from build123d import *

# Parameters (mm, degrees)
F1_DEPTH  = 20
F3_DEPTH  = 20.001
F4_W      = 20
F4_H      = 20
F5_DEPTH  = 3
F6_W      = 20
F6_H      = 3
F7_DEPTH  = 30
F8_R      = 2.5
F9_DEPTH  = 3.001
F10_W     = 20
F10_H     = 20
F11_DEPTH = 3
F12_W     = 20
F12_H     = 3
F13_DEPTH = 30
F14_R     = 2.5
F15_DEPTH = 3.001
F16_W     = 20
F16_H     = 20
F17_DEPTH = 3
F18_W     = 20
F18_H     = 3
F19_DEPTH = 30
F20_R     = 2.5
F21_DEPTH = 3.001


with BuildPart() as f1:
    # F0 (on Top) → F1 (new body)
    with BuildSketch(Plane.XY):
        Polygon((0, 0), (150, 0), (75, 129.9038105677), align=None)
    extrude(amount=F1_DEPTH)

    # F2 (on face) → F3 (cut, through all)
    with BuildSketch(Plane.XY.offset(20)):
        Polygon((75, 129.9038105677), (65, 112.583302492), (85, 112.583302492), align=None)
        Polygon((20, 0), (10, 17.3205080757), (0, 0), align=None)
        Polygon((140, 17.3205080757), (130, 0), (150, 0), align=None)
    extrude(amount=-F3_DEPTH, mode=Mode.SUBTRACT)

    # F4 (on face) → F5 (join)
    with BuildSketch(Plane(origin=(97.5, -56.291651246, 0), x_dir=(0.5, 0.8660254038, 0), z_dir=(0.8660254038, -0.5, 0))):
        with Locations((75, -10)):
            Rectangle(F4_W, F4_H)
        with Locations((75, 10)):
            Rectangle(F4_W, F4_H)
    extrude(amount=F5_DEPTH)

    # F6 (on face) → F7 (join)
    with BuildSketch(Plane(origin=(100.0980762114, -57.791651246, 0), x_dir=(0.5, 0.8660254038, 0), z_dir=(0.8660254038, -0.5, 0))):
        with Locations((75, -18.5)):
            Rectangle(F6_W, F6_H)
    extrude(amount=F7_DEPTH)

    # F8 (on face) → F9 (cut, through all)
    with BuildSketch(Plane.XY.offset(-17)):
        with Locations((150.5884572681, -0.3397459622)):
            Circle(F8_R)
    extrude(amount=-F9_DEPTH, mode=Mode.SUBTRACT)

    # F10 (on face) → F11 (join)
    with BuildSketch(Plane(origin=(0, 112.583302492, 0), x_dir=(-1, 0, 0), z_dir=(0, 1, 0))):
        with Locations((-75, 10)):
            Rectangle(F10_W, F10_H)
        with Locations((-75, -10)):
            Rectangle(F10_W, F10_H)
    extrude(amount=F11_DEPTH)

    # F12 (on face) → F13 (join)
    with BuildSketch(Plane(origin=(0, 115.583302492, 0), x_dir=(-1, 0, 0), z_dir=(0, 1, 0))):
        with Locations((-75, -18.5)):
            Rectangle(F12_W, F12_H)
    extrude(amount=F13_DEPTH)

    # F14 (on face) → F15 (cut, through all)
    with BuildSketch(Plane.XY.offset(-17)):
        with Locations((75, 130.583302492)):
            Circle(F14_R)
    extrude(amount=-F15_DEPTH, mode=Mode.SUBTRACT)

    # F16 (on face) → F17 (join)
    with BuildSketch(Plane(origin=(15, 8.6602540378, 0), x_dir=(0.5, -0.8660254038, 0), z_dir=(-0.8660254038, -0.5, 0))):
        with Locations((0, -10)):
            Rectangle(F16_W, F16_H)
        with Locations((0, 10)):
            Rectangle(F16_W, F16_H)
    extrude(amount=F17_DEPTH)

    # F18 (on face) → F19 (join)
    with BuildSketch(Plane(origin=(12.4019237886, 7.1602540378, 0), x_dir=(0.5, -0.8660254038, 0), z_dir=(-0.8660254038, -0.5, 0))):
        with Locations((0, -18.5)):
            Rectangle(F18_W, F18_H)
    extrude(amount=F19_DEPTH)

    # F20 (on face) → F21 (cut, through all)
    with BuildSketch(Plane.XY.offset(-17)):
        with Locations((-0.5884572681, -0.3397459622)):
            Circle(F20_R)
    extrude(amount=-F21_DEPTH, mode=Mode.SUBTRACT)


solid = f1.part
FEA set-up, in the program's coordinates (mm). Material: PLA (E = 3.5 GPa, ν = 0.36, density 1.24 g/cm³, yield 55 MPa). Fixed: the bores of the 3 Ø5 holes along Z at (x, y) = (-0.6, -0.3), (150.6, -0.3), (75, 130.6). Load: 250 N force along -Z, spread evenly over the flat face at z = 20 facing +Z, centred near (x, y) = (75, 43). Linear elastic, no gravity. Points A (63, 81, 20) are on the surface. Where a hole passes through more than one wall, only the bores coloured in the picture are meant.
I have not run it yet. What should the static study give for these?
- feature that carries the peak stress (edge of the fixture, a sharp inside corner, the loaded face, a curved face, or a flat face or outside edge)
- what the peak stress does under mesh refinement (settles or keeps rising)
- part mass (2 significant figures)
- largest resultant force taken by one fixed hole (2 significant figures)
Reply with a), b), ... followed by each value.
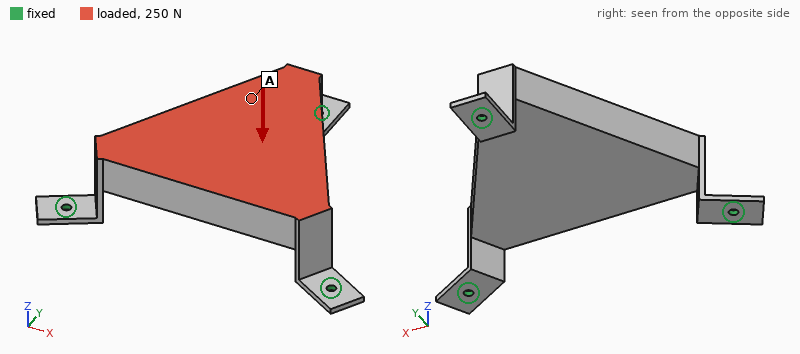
a) edge of the fixture
b) keeps rising
c) 240 g
d) 93 N
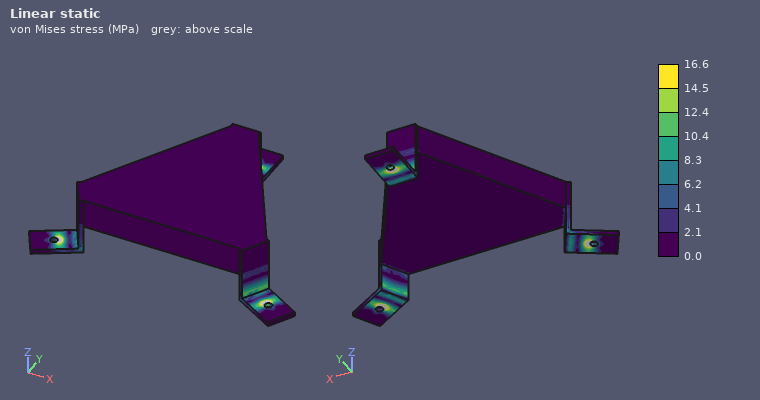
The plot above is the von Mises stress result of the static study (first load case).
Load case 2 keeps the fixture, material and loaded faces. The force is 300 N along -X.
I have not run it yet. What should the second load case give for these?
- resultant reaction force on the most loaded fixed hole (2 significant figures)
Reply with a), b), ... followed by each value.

a) 120 N
